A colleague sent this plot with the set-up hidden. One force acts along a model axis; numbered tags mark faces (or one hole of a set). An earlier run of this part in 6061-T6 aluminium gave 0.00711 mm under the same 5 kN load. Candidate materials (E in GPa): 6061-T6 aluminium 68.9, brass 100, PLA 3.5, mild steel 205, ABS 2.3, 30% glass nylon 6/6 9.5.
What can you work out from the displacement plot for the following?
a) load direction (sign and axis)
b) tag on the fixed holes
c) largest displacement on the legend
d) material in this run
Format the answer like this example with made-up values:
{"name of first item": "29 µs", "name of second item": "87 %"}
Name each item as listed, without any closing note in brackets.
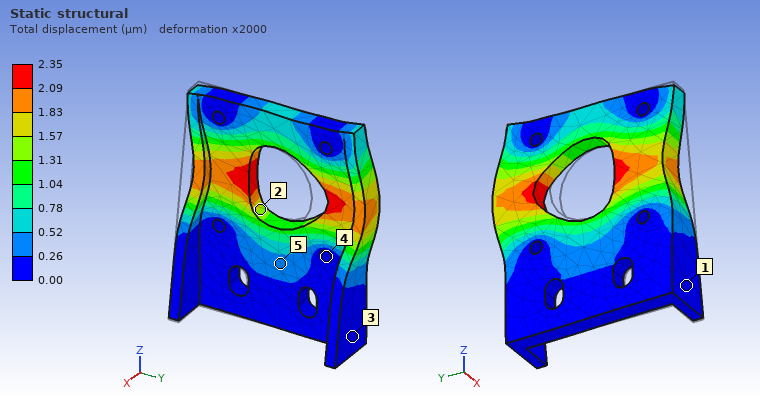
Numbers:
{"load direction": "+Y", "tag on the fixed holes": "4", "largest displacement on the legend": "2.35 µm", "material in this run": "mild steel"}
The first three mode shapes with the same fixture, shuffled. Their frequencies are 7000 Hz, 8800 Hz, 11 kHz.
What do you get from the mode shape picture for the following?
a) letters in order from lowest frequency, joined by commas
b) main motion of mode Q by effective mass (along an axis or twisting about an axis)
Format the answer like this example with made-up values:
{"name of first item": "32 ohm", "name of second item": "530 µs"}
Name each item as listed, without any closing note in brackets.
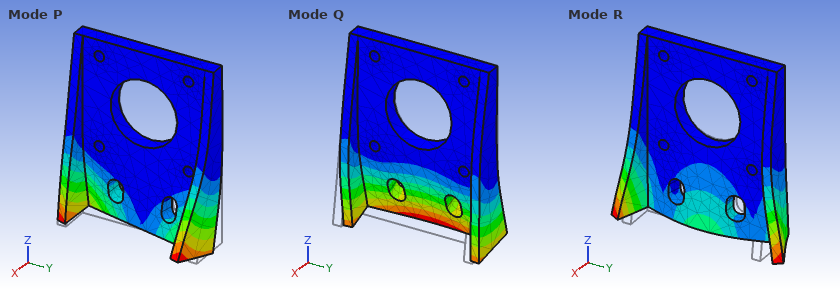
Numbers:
{"letters in order from lowest frequency, joined by commas": "Q, P, R", "main motion of mode Q by effective mass": "along X"}
